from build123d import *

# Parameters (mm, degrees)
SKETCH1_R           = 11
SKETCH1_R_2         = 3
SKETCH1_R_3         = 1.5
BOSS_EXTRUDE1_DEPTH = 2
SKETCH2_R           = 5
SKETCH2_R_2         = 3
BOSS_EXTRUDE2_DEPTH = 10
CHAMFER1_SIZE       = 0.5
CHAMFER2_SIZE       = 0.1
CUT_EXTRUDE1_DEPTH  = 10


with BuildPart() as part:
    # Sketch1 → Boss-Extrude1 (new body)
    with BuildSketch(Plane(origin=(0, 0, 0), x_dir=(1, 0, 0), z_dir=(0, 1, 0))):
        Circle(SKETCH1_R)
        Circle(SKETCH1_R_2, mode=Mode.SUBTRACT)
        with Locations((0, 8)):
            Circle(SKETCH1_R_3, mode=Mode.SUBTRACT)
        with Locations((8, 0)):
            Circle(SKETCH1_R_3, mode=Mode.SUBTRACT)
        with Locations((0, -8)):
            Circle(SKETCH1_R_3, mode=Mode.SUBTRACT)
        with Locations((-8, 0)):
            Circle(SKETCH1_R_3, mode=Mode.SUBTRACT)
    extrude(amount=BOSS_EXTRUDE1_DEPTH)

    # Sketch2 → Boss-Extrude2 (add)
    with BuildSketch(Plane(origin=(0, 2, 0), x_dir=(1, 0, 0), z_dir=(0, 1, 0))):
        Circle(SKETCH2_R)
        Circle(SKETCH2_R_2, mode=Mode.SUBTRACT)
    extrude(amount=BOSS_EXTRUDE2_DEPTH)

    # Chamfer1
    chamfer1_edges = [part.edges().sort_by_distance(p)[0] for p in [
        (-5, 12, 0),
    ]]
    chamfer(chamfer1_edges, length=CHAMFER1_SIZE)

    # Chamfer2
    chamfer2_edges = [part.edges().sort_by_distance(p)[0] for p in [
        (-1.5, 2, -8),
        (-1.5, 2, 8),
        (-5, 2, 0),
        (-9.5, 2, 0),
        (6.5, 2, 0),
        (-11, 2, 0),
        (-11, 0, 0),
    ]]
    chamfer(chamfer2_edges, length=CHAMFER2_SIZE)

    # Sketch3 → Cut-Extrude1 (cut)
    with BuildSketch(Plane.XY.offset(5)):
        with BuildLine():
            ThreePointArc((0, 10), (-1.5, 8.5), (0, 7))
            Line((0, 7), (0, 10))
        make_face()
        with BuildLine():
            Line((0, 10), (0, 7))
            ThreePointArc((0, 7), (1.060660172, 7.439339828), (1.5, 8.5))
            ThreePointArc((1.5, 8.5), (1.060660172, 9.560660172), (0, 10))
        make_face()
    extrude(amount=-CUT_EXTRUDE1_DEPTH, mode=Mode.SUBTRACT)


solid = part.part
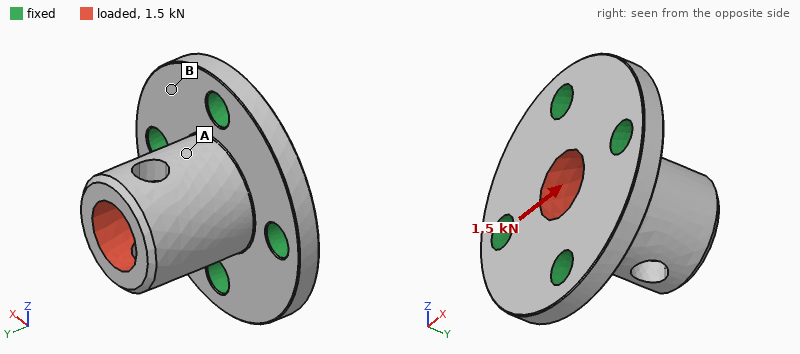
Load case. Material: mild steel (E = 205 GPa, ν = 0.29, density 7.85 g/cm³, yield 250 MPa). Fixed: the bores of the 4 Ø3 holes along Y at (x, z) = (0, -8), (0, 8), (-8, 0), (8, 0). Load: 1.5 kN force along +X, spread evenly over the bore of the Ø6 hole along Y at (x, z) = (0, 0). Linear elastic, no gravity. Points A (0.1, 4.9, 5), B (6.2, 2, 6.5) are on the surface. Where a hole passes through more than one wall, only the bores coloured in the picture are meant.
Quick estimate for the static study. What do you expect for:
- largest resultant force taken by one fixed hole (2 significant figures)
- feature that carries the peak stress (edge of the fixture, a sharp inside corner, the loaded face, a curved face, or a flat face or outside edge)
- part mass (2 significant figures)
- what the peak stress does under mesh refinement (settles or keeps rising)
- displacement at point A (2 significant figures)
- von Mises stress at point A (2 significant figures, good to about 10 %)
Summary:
740 N
edge of the fixture
8.8 g
keeps rising
3.7 µm
50 MPa
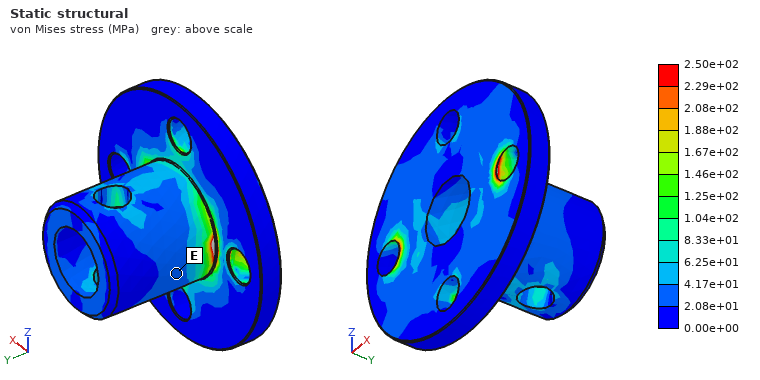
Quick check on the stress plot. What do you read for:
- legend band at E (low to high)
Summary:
2.08e+01 to 4.17e+01 MPa
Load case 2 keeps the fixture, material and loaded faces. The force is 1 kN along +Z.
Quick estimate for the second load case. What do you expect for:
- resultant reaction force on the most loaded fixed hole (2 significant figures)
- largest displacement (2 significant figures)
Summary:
490 N
7.4 µm
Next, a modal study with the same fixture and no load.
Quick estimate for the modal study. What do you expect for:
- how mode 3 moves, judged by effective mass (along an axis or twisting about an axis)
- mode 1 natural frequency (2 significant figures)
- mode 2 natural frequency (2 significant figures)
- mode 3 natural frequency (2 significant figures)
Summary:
along Y
31 kHz
32 kHz
54 kHz
